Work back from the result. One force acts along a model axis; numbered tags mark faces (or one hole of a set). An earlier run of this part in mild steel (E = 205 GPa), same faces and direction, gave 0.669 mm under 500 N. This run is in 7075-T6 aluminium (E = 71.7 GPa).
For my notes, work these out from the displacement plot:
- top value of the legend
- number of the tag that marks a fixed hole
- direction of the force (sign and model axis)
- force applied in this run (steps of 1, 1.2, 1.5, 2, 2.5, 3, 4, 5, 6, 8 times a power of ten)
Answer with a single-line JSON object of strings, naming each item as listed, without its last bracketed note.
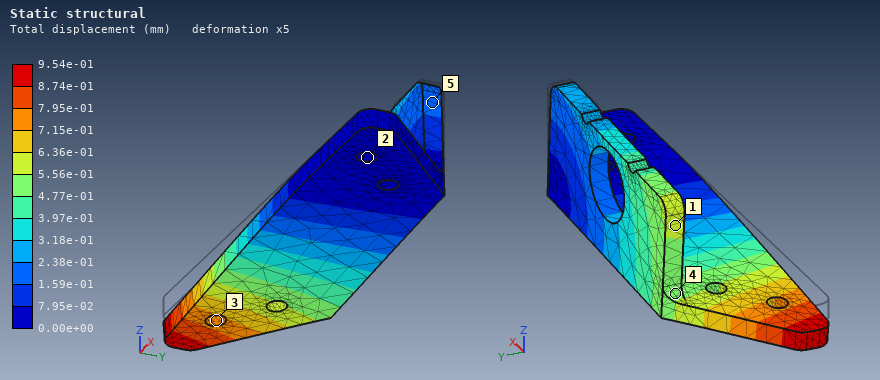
{"top value of the legend": "9.54e-01 mm", "number of the tag that marks a fixed hole": "2", "direction of the force": "-Z", "force applied in this run": "250 N"}
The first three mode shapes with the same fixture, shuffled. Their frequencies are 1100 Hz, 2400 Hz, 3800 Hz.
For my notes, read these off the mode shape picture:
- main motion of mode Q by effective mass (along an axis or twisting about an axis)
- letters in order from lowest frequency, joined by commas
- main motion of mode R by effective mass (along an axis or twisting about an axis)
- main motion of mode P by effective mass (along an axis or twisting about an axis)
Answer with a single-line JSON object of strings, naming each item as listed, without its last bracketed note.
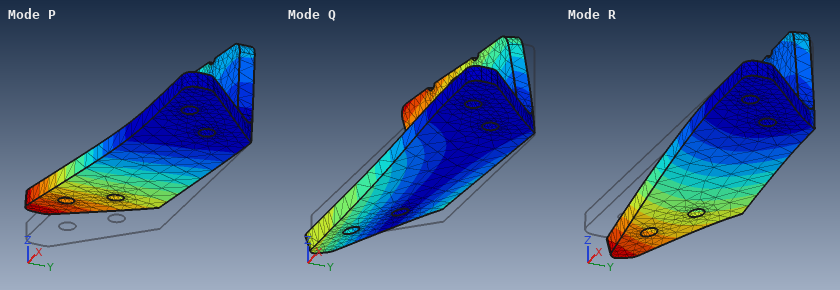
{"main motion of mode Q by effective mass": "along Y", "letters in order from lowest frequency, joined by commas": "P, Q, R", "main motion of mode R by effective mass": "along Y", "main motion of mode P by effective mass": "along Z"}
